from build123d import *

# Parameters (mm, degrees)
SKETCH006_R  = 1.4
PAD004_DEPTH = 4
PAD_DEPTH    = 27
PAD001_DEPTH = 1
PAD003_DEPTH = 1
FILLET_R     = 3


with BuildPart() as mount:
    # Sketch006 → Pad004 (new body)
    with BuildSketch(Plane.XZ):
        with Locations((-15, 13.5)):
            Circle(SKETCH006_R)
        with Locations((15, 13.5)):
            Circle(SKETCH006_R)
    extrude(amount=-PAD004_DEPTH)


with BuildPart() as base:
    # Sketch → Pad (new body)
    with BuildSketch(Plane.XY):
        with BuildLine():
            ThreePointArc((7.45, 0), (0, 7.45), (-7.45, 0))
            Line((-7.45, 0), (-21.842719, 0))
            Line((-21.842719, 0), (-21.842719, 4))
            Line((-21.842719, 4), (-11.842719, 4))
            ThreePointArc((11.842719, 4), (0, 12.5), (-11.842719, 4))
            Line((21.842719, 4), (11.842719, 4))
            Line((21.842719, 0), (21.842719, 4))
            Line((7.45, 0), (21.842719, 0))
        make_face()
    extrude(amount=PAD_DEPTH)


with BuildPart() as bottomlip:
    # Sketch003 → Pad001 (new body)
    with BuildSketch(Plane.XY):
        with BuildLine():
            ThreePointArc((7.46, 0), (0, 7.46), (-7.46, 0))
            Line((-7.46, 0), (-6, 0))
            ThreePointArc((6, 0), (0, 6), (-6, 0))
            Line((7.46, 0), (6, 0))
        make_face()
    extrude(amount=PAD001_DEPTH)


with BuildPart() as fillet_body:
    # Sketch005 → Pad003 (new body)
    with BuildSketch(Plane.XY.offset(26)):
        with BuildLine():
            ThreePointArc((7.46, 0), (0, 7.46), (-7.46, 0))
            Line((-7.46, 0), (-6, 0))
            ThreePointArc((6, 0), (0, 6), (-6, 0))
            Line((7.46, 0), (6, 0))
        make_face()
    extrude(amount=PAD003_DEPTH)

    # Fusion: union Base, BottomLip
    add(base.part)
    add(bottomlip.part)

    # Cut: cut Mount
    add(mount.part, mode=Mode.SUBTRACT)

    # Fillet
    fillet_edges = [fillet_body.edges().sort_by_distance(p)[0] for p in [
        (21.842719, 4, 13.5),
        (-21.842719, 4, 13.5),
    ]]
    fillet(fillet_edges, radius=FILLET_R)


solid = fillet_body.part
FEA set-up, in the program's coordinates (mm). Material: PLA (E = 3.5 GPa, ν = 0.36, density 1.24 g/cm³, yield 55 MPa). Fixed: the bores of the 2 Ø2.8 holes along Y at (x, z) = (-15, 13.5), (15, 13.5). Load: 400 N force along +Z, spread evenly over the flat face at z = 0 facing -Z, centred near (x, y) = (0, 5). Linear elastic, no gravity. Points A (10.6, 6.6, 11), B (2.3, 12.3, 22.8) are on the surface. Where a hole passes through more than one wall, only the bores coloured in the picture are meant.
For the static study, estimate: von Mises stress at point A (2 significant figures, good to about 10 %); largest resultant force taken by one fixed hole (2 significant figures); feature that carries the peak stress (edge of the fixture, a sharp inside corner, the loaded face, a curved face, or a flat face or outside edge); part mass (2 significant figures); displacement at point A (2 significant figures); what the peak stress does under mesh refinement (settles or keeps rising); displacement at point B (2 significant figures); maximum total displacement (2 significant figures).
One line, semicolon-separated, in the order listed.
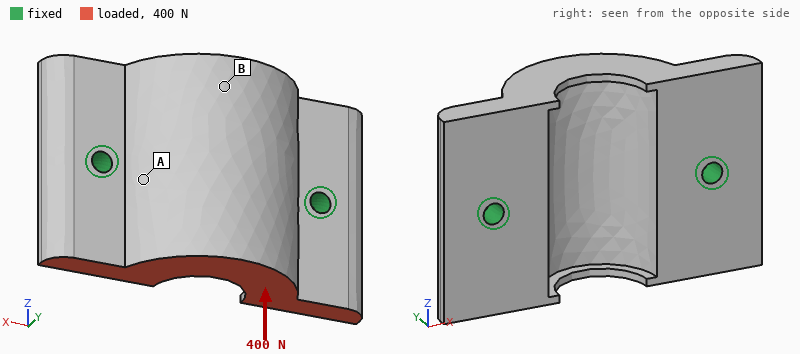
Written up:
5.7 MPa; 200 N; edge of the fixture; 7.7 g; 0.053 mm; keeps rising; 0.13 mm; 0.16 mm
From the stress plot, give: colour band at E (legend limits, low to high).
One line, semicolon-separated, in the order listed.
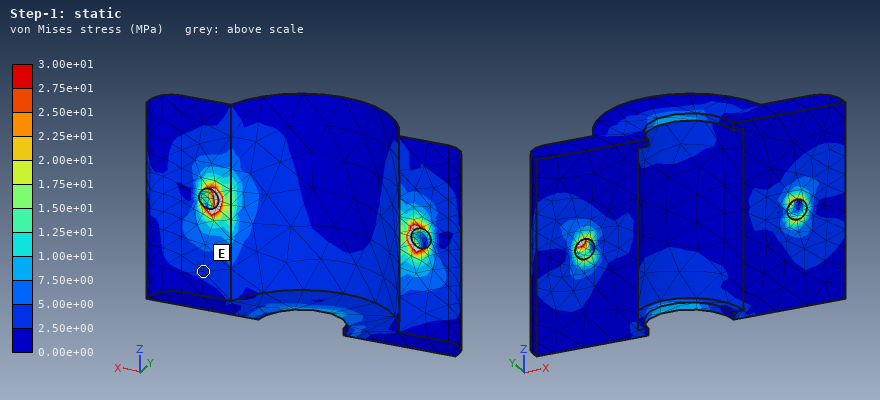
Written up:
2.50e+00 to 5.00e+00 MPa
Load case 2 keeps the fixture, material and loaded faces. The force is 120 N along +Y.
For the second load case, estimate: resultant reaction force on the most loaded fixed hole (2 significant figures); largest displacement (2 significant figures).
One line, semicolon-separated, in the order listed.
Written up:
71 N; 0.18 mm
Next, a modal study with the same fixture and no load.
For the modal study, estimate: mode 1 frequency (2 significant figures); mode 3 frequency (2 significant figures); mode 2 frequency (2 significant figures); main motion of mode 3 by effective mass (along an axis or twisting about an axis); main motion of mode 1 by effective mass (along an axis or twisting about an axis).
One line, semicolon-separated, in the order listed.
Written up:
2700 Hz; 6500 Hz; 6000 Hz; along Y; along Z
